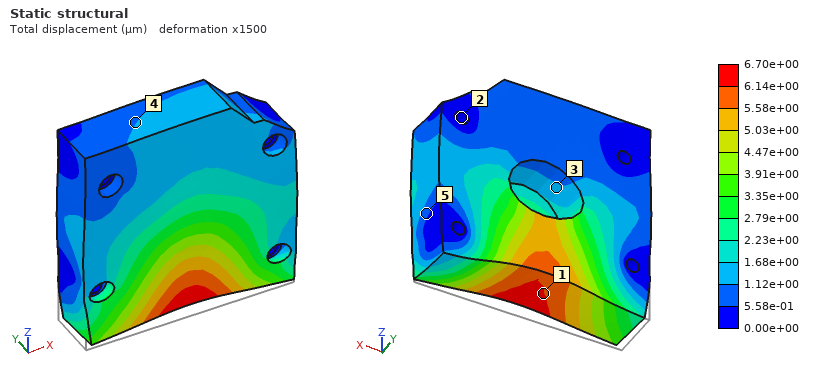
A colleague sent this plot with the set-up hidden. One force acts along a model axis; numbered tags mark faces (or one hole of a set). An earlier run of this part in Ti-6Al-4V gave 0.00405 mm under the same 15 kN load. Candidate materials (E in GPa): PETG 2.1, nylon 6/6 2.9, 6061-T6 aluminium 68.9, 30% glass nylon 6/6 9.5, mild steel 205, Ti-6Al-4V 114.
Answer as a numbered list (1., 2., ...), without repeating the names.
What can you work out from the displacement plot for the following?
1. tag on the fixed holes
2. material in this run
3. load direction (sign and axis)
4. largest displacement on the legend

1. 2
2. 6061-T6 aluminium
3. +Z
4. 6.70e+00 µm
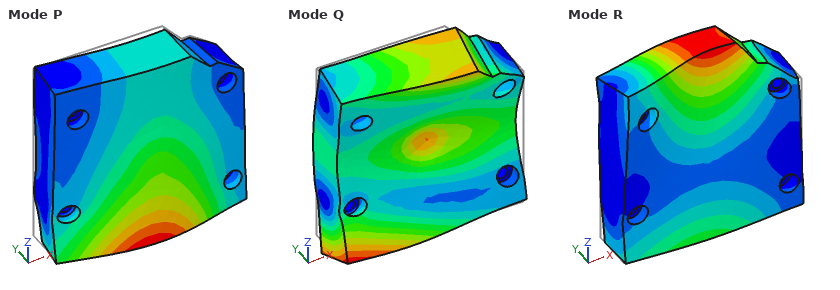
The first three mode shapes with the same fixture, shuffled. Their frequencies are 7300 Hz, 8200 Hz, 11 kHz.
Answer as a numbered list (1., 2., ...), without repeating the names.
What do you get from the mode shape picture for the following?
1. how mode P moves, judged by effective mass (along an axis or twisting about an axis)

1. along Y
